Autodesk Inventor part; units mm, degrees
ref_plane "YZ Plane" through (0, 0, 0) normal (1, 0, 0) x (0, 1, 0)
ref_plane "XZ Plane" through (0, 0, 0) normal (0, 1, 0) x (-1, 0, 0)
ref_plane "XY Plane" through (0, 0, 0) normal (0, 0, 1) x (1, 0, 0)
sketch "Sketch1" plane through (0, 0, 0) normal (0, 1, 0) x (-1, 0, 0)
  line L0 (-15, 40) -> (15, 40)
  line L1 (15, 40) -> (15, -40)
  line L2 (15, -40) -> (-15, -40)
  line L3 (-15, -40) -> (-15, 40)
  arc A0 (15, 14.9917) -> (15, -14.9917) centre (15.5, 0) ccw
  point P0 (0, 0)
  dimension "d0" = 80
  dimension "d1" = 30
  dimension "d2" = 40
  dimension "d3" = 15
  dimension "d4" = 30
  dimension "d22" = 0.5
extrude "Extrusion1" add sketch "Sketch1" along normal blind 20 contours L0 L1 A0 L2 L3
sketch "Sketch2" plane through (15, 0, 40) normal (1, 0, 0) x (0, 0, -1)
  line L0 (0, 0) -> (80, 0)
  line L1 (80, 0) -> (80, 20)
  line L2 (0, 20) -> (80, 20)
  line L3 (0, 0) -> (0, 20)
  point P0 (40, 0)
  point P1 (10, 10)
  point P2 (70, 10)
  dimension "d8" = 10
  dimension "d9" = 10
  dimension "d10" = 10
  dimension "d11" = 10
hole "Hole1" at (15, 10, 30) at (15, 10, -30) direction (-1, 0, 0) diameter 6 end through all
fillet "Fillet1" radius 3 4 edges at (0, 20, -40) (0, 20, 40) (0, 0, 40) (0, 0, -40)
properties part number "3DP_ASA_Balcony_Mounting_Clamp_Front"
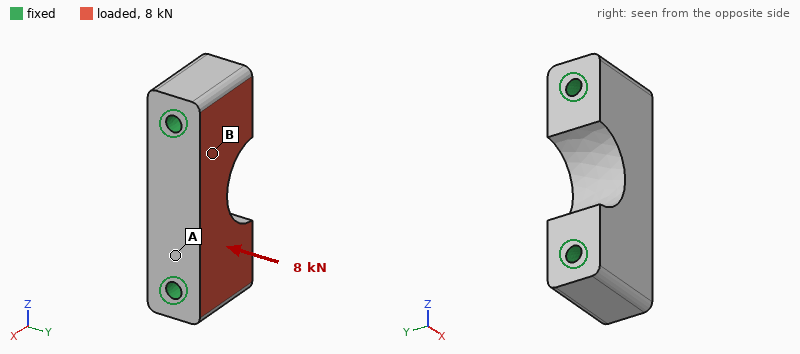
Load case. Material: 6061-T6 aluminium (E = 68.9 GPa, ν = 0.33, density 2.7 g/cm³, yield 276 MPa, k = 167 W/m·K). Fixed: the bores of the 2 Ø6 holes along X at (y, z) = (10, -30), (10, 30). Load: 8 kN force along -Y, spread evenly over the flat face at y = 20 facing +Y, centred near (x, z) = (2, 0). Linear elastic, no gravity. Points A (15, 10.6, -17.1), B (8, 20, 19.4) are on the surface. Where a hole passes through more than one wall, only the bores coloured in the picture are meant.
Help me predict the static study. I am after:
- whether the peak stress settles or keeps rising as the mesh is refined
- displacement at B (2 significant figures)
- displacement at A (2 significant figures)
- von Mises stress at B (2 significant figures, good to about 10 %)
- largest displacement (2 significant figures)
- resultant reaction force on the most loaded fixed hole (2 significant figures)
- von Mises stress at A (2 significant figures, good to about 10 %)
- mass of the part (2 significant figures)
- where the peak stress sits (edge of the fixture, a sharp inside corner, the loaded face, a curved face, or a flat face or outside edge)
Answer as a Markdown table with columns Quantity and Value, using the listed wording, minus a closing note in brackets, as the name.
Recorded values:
| Quantity | Value |
|---|---|
| whether the peak stress settles or keeps rising as the mesh is refined | keeps rising |
| displacement at B | 5.4 µm |
| displacement at A | 5.7 µm |
| von Mises stress at B | 4.8 MPa |
| largest displacement | 10 µm |
| resultant reaction force on the most loaded fixed hole | 4.0 kN |
| von Mises stress at A | 11 MPa |
| mass of the part | 110 g |
| where the peak stress sits | edge of the fixture |
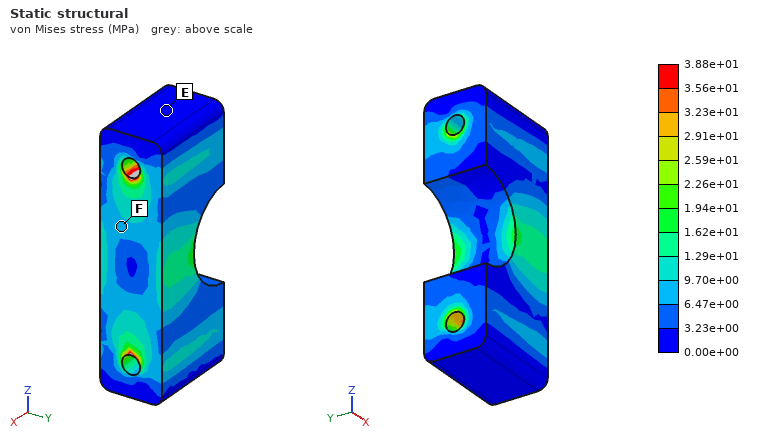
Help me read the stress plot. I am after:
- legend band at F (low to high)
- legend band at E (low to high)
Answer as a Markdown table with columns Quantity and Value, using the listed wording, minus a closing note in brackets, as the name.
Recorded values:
| Quantity | Value |
|---|---|
| legend band at F | 6.47e+00 to 9.70e+00 MPa |
| legend band at E | 0.00e+00 to 3.23e+00 MPa |
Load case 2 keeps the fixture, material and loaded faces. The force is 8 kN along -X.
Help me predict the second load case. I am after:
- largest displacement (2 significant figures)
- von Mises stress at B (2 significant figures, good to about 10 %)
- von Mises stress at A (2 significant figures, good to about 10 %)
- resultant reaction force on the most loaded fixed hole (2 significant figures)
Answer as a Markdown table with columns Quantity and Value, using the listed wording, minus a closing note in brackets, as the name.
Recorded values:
| Quantity | Value |
|---|---|
| largest displacement | 12 µm |
| von Mises stress at B | 17 MPa |
| von Mises stress at A | 10 MPa |
| resultant reaction force on the most loaded fixed hole | 4.0 kN |
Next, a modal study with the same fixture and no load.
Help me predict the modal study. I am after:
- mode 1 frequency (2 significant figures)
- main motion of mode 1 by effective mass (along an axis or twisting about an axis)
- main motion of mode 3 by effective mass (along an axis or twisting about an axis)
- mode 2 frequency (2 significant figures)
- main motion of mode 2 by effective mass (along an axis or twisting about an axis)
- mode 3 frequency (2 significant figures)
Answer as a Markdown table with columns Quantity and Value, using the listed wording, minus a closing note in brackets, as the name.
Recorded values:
| Quantity | Value |
|---|---|
| mode 1 frequency | 16 kHz |
| main motion of mode 1 by effective mass | along Y |
| main motion of mode 3 by effective mass | twisting about Z |
| mode 2 frequency | 24 kHz |
| main motion of mode 2 by effective mass | along X |
| mode 3 frequency | 31 kHz |
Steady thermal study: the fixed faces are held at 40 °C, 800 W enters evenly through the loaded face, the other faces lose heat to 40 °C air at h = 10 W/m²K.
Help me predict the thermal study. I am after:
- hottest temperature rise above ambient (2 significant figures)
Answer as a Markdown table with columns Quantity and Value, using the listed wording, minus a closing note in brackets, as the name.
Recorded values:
| Quantity | Value |
|---|---|
| hottest temperature rise above ambient | 66 K |
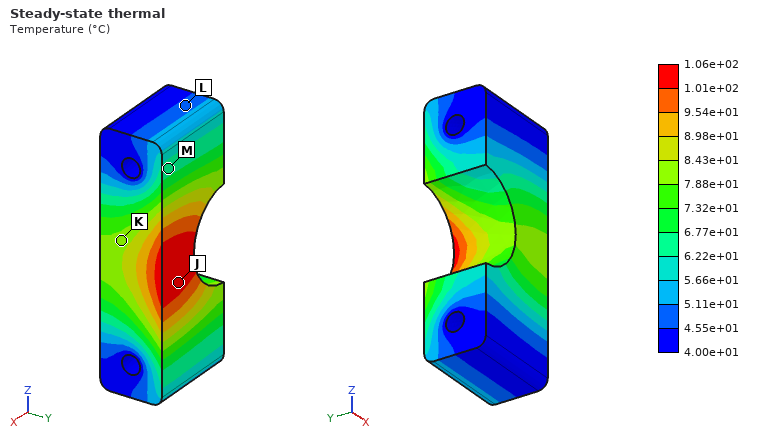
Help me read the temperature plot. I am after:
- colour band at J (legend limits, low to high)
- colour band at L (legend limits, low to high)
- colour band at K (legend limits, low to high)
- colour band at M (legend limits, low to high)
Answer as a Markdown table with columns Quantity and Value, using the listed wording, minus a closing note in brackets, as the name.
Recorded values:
| Quantity | Value |
|---|---|
| colour band at J | 1.01e+02 to 1.06e+02 °C |
| colour band at L | 4.55e+01 to 5.11e+01 °C |
| colour band at K | 7.88e+01 to 8.43e+01 °C |
| colour band at M | 6.22e+01 to 6.77e+01 °C |
